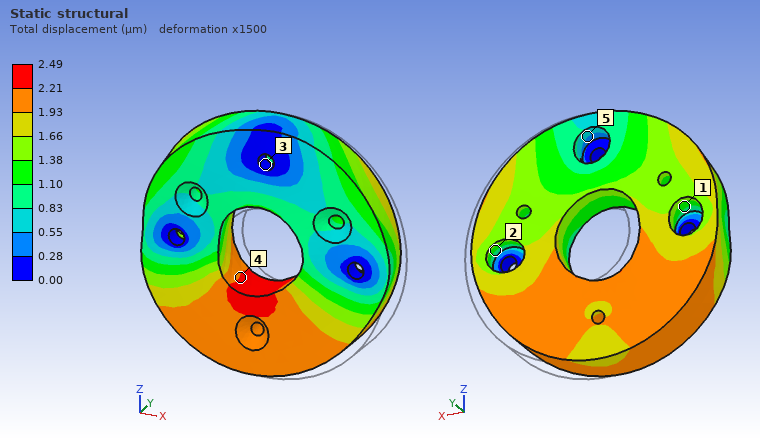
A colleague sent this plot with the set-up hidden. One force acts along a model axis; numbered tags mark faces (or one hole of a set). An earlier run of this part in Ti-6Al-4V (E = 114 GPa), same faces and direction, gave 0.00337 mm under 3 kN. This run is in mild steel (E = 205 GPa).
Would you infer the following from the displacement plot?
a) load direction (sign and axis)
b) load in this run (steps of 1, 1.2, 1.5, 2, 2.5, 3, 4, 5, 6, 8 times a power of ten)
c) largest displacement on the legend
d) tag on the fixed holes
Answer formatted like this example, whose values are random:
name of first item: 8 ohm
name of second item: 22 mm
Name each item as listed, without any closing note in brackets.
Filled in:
load direction: -X
load in this run: 4 kN
largest displacement on the legend: 2.49 µm
tag on the fixed holes: 3
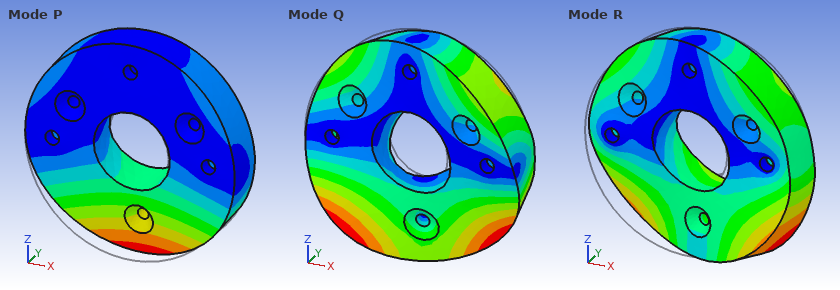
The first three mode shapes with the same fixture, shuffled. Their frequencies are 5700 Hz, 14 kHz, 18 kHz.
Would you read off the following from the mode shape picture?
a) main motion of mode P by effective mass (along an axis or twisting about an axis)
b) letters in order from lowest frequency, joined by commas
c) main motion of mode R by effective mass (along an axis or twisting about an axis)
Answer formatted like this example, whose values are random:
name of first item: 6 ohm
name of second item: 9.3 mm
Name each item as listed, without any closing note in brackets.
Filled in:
main motion of mode P by effective mass: along Y
letters in order from lowest frequency, joined by commas: P, Q, R
main motion of mode R by effective mass: along X
